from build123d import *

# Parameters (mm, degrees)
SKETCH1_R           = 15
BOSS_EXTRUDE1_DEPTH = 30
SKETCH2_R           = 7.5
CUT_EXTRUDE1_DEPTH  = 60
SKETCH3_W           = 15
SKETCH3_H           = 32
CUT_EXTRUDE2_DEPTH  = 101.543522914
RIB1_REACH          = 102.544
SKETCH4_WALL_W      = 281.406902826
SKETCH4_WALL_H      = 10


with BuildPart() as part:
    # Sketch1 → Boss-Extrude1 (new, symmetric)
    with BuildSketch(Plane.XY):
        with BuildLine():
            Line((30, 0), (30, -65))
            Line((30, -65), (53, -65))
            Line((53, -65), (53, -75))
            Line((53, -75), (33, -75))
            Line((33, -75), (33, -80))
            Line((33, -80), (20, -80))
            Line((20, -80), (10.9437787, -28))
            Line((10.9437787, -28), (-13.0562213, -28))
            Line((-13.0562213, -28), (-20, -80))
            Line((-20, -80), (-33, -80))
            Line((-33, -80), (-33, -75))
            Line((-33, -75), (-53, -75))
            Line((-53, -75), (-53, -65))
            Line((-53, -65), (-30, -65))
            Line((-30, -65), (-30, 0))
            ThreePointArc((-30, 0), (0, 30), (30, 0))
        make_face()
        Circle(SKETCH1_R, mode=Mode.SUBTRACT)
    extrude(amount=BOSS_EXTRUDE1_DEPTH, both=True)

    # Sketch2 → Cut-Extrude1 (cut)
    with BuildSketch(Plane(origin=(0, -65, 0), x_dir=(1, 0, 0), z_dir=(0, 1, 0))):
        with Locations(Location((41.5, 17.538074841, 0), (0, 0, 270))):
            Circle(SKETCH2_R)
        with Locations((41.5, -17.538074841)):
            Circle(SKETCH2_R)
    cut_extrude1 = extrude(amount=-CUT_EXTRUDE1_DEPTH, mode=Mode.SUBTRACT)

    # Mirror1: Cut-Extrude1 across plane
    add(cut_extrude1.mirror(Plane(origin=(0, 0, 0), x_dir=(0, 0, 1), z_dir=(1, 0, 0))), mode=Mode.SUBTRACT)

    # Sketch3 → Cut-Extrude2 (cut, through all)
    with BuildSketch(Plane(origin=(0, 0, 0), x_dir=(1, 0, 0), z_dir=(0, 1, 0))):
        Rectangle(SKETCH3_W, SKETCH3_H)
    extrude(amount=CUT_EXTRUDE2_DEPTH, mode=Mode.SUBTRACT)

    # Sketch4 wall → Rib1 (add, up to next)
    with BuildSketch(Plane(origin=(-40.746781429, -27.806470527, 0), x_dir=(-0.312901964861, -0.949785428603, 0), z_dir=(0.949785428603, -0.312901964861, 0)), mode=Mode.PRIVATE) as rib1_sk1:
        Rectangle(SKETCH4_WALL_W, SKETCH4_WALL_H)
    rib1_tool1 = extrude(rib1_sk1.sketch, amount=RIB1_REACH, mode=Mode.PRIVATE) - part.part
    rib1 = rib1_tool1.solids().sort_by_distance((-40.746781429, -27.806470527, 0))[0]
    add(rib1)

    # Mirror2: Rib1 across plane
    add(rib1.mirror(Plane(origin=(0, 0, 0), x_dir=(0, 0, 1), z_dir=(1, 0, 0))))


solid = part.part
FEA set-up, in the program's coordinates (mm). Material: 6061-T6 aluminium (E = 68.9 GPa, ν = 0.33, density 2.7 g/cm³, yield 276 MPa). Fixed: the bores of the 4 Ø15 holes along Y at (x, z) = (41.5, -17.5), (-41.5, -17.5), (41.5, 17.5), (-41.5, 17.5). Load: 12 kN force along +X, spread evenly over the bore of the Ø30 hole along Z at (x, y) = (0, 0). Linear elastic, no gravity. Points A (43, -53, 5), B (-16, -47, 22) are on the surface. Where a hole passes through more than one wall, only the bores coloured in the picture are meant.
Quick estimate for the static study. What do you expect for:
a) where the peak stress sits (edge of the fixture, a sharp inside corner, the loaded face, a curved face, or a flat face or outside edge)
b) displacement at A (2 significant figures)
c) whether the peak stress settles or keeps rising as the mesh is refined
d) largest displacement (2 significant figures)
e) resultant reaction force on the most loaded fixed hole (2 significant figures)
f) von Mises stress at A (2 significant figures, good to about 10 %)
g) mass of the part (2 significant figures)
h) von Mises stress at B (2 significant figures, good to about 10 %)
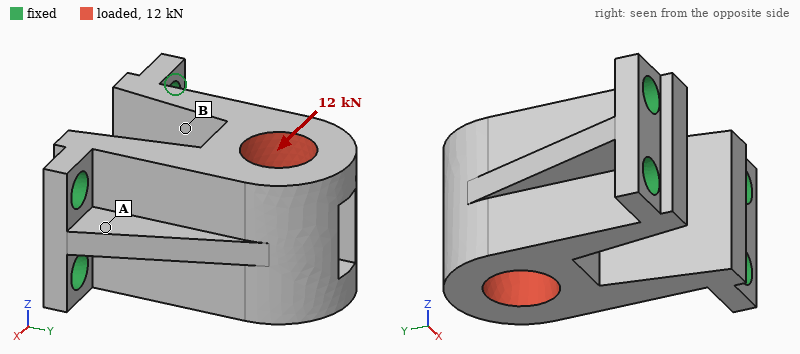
edge of the fixture
19 µm
keeps rising
76 µm
6.0 kN
27 MPa
710 g
10 MPa
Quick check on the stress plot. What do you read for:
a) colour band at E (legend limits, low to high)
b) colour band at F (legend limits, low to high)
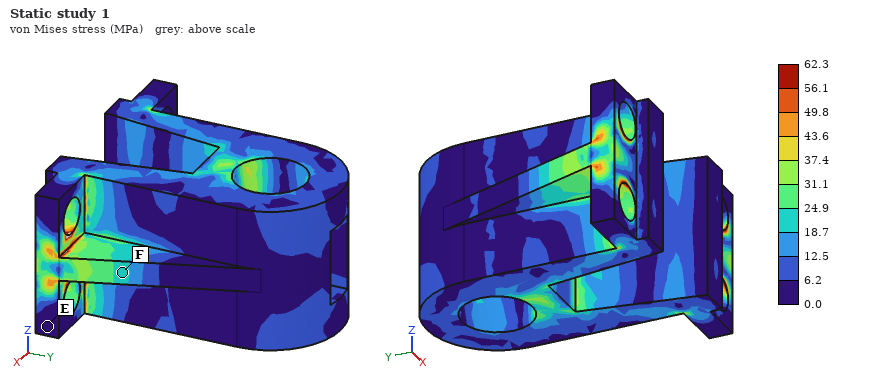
0.0 to 6.2 MPa
18.7 to 24.9 MPa
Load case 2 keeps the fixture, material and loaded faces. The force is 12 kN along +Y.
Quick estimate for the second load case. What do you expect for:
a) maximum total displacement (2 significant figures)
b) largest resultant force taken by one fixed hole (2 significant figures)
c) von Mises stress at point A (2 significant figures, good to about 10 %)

12 µm
3.2 kN
9.4 MPa
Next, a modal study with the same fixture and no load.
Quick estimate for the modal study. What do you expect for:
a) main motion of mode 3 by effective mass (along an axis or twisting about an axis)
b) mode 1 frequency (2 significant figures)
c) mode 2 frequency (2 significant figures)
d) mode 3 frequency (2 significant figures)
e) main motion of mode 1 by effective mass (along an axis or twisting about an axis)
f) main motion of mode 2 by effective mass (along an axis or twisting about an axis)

twisting about Y
2300 Hz
3500 Hz
4400 Hz
along Z
along X
